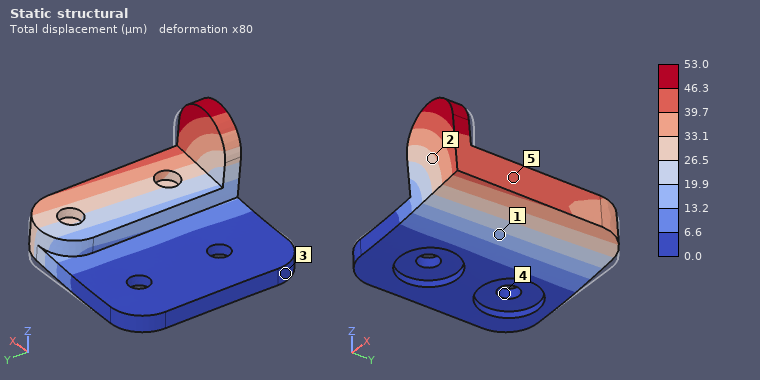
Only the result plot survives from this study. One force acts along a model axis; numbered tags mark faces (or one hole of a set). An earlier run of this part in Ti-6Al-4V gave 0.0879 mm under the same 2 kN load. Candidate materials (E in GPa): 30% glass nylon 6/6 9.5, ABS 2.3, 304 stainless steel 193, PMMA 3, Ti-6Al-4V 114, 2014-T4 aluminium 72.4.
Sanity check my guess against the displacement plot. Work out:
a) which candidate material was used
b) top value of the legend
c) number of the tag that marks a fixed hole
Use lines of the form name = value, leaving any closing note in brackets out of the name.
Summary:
which candidate material was used = 304 stainless steel
top value of the legend = 53.0 µm
number of the tag that marks a fixed hole = 4
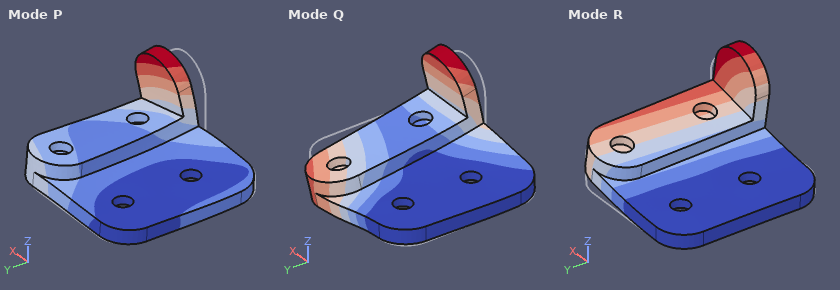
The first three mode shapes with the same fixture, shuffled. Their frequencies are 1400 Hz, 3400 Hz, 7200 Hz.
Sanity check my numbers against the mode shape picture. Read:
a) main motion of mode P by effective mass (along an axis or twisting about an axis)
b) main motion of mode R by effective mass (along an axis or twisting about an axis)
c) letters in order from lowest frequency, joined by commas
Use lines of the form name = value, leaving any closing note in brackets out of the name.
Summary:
main motion of mode P by effective mass = along Y
main motion of mode R by effective mass = along Z
letters in order from lowest frequency, joined by commas = R, Q, P
